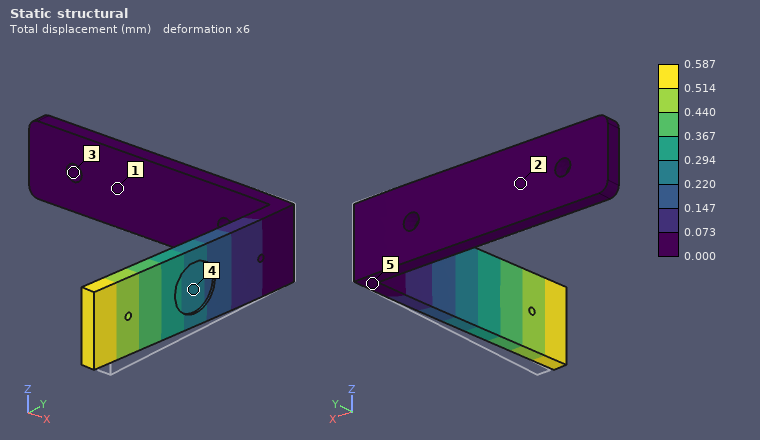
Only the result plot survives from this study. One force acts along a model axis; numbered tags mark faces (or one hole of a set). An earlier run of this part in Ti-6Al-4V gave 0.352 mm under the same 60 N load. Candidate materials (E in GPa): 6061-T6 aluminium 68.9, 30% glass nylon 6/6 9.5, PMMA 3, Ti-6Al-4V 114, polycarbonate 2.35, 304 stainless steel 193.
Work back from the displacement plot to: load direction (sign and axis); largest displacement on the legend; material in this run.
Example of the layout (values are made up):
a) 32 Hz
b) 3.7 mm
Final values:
a) -X
b) 0.587 mm
c) 6061-T6 aluminium
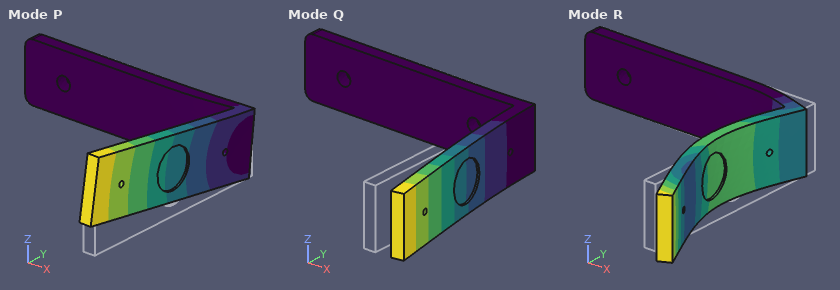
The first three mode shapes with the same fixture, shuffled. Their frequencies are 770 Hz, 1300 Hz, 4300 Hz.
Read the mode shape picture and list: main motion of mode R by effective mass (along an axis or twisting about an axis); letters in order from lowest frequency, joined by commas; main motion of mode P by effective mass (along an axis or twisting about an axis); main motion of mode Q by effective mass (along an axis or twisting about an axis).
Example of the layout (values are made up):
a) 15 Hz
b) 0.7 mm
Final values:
a) along Y
b) Q, P, R
c) along Z
d) along X
